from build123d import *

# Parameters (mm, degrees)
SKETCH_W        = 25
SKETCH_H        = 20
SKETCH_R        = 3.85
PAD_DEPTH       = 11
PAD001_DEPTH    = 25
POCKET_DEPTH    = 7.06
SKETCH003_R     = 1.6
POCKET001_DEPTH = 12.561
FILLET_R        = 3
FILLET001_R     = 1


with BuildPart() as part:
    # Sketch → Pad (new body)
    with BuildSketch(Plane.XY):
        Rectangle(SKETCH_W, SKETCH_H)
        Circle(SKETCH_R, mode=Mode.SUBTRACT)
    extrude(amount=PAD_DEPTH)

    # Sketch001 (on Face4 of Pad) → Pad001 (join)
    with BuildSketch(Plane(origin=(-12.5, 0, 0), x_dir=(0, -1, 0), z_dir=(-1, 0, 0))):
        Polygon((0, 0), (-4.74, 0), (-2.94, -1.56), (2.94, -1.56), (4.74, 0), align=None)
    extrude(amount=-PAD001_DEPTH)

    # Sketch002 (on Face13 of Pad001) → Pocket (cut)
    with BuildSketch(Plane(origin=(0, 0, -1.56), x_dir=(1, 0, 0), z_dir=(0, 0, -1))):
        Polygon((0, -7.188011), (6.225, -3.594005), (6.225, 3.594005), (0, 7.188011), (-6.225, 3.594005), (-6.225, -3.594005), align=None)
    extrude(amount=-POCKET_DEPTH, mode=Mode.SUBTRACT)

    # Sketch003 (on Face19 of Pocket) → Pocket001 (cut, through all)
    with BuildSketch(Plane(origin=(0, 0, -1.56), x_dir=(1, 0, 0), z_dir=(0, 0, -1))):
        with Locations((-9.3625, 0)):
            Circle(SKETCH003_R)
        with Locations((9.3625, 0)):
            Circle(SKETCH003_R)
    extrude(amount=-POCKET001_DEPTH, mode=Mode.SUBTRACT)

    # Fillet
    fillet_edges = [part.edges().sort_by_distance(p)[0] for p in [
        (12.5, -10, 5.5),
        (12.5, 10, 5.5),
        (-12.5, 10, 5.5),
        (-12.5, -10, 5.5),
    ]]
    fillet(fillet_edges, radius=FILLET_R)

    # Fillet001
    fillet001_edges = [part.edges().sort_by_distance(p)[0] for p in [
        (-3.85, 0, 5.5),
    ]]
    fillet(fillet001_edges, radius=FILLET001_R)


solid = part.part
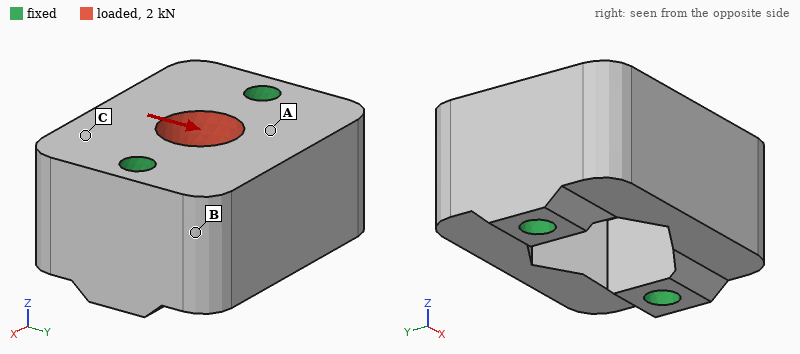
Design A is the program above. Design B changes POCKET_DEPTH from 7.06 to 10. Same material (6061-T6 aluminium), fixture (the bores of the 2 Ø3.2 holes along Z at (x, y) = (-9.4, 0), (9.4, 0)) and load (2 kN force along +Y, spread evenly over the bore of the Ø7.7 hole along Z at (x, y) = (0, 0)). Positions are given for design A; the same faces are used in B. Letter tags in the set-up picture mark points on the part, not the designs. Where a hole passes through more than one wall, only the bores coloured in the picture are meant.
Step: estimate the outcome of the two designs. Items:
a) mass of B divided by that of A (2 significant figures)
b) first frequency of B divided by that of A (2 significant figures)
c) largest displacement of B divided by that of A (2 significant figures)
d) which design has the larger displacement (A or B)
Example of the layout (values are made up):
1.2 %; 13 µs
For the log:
0.94; 1.00; 1.9; B
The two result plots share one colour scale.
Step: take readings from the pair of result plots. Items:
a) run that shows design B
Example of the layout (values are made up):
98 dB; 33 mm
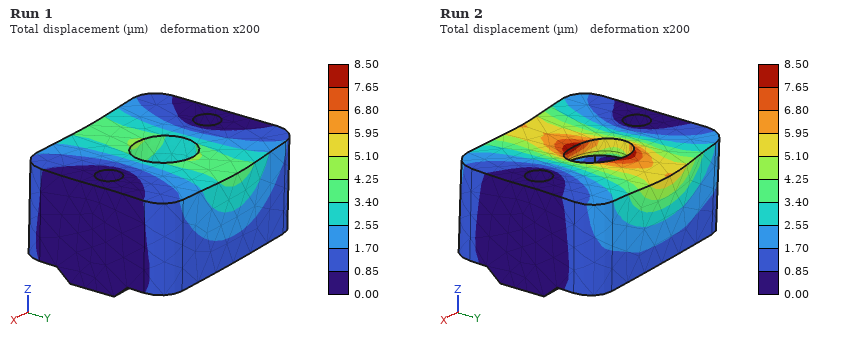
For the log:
Run 2
